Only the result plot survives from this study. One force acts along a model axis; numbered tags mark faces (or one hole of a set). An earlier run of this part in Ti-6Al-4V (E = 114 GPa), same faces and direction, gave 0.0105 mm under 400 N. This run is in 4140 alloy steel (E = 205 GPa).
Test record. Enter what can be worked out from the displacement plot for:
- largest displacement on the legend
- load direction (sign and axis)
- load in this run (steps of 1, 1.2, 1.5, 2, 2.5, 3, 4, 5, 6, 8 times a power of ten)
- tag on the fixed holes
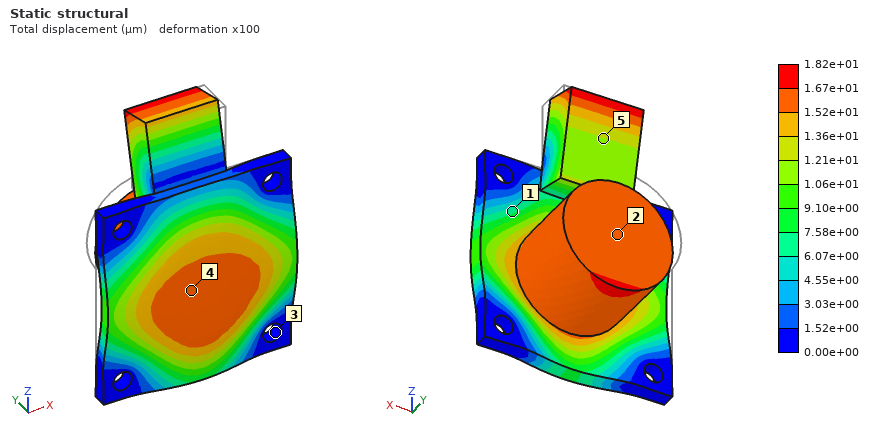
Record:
1.82e+01 µm
-Y
1.2 kN
3
